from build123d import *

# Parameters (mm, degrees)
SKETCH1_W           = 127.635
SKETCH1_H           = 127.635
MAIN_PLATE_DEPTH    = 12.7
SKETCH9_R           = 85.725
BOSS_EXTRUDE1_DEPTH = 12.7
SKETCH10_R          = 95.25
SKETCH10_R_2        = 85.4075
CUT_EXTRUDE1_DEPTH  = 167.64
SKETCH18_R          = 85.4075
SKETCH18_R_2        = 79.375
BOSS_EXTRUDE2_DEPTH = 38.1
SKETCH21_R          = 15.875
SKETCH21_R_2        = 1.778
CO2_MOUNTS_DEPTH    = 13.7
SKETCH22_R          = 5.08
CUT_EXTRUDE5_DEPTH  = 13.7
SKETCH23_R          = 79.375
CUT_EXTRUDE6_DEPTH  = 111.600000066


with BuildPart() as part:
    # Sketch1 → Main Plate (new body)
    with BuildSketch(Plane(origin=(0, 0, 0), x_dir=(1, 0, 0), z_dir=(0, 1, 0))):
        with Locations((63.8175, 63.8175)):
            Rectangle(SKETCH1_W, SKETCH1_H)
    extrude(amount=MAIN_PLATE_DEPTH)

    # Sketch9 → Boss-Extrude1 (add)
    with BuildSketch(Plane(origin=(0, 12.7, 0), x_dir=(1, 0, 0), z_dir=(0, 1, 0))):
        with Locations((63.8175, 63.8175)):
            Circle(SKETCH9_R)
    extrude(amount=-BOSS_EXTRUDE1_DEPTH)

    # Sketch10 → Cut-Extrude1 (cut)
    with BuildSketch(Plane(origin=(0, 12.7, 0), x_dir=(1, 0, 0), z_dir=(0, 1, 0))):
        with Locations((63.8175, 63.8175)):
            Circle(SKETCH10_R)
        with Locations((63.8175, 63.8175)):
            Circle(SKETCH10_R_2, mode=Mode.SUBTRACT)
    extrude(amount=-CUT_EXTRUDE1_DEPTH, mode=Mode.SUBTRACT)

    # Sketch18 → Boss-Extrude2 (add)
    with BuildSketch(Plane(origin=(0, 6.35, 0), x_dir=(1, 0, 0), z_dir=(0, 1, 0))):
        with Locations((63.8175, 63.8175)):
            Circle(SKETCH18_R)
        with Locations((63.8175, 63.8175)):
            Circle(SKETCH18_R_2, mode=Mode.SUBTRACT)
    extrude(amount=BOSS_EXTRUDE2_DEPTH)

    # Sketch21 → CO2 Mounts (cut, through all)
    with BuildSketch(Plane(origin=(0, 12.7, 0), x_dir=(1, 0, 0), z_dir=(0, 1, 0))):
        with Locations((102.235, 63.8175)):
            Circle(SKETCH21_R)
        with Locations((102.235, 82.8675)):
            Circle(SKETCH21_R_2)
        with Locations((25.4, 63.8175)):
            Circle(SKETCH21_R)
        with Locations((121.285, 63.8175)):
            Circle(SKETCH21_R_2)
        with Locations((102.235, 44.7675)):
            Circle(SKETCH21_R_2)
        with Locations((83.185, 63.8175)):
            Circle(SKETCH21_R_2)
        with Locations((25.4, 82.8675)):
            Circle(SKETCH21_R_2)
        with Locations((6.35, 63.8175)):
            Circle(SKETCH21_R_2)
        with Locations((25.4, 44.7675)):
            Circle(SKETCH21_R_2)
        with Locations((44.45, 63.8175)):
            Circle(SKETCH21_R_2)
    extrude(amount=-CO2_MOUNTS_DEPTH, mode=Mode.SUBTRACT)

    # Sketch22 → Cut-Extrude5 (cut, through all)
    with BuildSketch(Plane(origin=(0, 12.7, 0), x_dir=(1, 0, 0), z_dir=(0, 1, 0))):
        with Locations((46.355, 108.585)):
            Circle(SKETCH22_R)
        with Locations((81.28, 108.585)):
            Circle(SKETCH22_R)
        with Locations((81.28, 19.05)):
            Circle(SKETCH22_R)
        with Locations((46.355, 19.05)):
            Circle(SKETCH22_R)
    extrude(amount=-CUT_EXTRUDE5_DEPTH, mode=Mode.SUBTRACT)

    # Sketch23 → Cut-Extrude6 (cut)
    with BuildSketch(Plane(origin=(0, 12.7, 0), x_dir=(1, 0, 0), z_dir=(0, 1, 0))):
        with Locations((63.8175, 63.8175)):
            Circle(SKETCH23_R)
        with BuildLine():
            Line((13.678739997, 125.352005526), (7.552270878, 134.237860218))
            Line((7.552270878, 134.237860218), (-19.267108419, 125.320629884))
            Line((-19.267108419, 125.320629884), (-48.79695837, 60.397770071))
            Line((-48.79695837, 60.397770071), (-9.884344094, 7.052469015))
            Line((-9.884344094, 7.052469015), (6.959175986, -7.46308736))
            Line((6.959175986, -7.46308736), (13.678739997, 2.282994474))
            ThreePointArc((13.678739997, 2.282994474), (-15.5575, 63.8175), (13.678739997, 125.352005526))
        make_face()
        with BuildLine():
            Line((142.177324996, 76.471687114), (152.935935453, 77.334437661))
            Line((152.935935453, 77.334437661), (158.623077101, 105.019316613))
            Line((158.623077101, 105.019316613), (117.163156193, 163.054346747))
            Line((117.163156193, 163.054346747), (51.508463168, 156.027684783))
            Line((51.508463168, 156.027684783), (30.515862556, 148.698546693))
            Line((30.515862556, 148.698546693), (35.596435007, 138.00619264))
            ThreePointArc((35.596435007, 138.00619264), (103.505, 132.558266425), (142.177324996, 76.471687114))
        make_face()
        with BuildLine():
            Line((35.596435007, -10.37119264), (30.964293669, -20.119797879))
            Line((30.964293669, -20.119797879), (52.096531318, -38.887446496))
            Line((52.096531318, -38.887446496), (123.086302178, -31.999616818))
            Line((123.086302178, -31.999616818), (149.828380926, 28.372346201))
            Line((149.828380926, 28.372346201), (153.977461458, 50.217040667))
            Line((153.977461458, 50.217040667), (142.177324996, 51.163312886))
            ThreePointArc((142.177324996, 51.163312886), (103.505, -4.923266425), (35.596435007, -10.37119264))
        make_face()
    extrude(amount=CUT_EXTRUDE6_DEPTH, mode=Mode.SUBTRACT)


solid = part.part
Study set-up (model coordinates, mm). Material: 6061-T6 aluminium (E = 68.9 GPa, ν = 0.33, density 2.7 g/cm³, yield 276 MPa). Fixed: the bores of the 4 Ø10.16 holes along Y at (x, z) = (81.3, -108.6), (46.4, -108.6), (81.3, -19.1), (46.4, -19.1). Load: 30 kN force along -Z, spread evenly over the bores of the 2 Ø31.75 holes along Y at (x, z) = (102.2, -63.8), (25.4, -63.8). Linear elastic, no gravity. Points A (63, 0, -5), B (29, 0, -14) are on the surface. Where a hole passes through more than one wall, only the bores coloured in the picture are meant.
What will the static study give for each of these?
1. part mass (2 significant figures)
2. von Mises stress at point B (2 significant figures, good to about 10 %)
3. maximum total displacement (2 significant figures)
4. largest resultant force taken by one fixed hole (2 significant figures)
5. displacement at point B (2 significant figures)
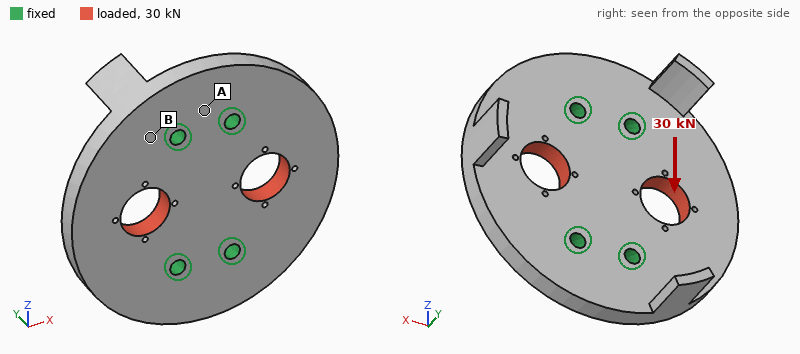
760 g
10 MPa
18 µm
7.5 kN
6.0 µm
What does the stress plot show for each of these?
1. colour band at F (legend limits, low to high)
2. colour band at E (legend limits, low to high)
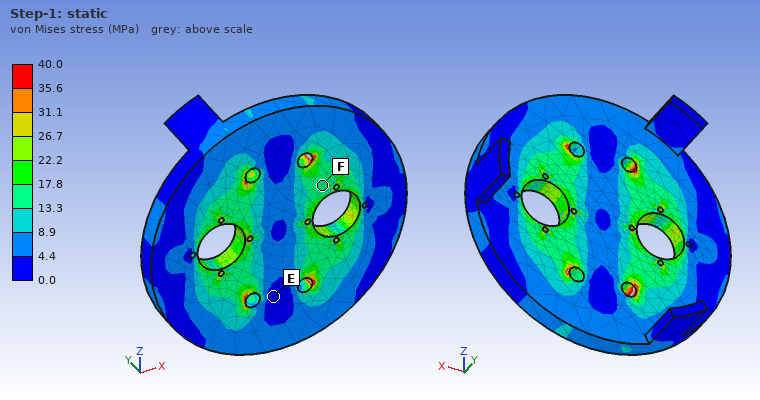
13.3 to 17.8 MPa
0.0 to 4.4 MPa
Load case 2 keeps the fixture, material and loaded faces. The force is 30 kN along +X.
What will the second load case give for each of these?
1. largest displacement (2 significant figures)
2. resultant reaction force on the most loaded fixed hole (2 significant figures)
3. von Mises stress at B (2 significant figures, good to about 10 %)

18 µm
7.5 kN
9.1 MPa
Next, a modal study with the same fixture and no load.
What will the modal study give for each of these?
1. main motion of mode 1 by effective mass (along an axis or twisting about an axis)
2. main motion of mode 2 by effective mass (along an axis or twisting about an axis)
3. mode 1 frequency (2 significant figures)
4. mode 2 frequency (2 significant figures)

along Y
along Y
2100 Hz
2400 Hz
